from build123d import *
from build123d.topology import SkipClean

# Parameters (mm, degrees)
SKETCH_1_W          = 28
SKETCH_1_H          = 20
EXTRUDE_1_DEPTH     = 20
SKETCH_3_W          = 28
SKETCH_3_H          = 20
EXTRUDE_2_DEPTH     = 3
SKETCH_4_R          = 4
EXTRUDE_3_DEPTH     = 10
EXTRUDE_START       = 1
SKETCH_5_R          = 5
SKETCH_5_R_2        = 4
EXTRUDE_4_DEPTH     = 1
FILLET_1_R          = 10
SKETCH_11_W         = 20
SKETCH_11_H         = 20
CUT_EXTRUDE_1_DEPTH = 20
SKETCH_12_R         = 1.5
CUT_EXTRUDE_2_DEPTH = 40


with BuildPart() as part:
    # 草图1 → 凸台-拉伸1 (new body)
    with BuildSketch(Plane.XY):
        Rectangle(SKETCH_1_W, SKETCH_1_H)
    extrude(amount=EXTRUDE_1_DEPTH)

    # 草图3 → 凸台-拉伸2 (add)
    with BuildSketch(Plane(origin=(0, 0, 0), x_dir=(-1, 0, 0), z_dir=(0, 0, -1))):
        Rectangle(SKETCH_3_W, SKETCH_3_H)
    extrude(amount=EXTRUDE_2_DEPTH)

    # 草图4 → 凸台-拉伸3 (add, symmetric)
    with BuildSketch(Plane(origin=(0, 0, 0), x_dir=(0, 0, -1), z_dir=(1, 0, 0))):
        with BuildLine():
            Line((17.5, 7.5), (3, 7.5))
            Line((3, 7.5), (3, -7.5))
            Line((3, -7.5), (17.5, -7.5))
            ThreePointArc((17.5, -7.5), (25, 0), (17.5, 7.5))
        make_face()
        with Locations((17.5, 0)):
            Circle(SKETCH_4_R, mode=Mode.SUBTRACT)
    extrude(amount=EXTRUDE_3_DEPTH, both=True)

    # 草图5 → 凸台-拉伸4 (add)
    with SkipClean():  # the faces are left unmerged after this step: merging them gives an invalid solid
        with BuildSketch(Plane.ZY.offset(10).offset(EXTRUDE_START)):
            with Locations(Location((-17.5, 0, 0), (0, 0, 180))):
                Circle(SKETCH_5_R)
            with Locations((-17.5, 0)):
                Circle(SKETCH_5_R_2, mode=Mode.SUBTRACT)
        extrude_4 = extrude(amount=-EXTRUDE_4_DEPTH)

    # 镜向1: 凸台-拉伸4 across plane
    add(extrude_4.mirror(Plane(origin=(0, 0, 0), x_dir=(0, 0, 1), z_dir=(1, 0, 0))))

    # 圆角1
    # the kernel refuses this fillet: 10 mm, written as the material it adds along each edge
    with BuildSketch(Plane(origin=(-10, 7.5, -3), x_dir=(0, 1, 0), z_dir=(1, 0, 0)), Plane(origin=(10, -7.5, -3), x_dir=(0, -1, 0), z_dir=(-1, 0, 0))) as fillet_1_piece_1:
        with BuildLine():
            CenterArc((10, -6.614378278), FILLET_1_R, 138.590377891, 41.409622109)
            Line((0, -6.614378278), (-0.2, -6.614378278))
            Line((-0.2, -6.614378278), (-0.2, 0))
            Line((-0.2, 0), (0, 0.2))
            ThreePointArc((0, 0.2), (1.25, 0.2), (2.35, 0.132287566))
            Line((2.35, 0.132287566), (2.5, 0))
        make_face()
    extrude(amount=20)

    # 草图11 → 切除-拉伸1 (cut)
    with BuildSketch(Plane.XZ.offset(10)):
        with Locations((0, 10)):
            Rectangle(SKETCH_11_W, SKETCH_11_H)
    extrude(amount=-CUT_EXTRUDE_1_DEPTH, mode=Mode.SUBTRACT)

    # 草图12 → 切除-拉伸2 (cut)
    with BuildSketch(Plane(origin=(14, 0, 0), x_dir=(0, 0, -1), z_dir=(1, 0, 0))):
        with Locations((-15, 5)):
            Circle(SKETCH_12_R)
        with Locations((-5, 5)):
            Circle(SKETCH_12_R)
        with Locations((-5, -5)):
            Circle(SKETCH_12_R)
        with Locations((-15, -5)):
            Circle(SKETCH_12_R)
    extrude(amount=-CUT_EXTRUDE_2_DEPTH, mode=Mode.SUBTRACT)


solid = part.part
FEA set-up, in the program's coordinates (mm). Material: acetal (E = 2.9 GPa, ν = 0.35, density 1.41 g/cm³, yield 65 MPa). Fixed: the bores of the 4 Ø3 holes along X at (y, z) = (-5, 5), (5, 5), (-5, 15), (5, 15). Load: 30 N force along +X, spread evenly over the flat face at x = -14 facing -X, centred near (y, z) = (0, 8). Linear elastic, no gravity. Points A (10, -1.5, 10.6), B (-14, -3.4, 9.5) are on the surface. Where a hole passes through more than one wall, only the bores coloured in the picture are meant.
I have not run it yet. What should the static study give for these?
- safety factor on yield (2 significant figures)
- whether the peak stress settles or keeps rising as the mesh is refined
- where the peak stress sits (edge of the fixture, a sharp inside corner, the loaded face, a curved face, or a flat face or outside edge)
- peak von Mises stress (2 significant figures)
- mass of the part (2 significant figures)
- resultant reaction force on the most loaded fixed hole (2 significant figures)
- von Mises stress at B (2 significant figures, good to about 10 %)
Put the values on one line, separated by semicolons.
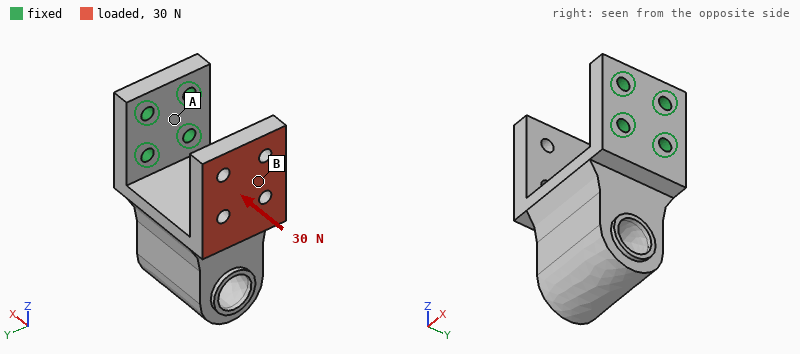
9.6; settles; a curved face; 6.8 MPa; 14 g; 14 N; 1.2 MPa
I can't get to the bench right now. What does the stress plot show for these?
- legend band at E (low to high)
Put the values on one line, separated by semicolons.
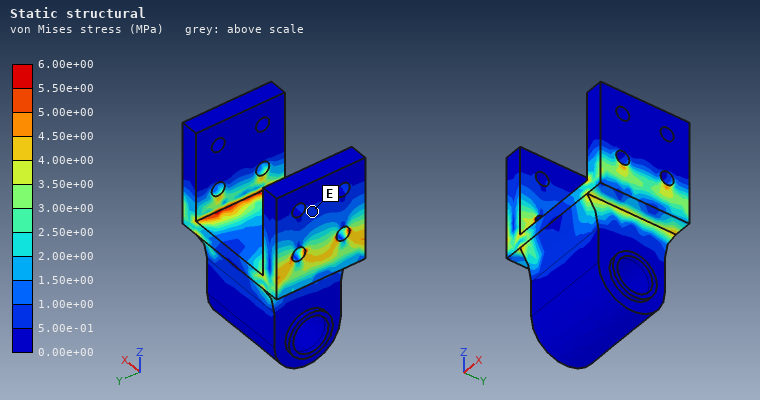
5.00e-01 to 1.00e+00 MPa
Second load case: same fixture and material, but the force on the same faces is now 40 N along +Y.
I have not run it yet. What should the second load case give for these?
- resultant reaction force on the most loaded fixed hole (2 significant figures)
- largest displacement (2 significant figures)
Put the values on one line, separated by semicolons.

83 N; 0.35 mm
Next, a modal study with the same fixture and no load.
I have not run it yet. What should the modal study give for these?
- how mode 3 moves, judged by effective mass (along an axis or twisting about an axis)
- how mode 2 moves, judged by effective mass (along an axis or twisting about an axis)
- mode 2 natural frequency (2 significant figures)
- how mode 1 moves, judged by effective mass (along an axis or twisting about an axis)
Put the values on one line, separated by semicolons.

along X; along Y; 1100 Hz; along Z
